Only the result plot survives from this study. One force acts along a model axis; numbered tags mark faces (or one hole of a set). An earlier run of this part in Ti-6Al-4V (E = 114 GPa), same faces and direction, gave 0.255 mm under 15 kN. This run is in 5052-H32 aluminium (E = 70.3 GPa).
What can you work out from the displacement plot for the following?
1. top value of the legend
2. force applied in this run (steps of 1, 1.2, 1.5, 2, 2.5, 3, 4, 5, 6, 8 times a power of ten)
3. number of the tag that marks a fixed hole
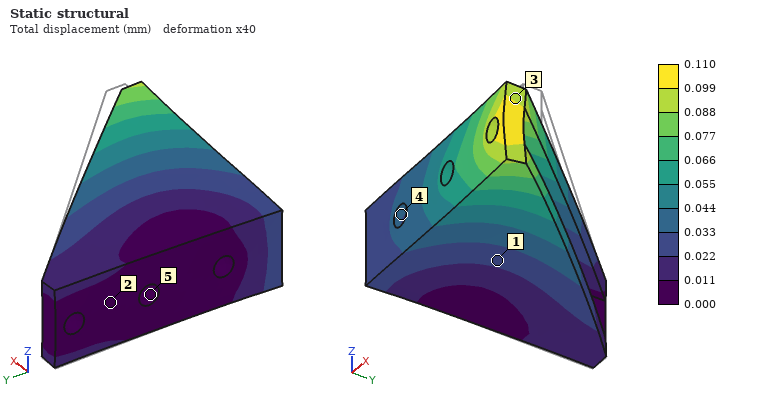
0.110 mm
4 kN
5
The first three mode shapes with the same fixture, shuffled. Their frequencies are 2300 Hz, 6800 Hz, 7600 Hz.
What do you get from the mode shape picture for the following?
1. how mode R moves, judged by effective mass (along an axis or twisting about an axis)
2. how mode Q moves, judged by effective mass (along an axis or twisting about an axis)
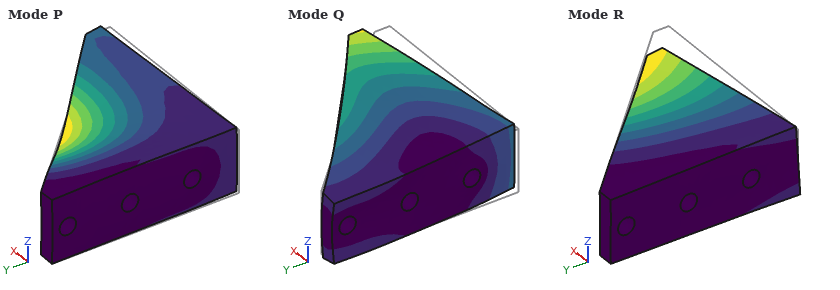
along Z
along Y
